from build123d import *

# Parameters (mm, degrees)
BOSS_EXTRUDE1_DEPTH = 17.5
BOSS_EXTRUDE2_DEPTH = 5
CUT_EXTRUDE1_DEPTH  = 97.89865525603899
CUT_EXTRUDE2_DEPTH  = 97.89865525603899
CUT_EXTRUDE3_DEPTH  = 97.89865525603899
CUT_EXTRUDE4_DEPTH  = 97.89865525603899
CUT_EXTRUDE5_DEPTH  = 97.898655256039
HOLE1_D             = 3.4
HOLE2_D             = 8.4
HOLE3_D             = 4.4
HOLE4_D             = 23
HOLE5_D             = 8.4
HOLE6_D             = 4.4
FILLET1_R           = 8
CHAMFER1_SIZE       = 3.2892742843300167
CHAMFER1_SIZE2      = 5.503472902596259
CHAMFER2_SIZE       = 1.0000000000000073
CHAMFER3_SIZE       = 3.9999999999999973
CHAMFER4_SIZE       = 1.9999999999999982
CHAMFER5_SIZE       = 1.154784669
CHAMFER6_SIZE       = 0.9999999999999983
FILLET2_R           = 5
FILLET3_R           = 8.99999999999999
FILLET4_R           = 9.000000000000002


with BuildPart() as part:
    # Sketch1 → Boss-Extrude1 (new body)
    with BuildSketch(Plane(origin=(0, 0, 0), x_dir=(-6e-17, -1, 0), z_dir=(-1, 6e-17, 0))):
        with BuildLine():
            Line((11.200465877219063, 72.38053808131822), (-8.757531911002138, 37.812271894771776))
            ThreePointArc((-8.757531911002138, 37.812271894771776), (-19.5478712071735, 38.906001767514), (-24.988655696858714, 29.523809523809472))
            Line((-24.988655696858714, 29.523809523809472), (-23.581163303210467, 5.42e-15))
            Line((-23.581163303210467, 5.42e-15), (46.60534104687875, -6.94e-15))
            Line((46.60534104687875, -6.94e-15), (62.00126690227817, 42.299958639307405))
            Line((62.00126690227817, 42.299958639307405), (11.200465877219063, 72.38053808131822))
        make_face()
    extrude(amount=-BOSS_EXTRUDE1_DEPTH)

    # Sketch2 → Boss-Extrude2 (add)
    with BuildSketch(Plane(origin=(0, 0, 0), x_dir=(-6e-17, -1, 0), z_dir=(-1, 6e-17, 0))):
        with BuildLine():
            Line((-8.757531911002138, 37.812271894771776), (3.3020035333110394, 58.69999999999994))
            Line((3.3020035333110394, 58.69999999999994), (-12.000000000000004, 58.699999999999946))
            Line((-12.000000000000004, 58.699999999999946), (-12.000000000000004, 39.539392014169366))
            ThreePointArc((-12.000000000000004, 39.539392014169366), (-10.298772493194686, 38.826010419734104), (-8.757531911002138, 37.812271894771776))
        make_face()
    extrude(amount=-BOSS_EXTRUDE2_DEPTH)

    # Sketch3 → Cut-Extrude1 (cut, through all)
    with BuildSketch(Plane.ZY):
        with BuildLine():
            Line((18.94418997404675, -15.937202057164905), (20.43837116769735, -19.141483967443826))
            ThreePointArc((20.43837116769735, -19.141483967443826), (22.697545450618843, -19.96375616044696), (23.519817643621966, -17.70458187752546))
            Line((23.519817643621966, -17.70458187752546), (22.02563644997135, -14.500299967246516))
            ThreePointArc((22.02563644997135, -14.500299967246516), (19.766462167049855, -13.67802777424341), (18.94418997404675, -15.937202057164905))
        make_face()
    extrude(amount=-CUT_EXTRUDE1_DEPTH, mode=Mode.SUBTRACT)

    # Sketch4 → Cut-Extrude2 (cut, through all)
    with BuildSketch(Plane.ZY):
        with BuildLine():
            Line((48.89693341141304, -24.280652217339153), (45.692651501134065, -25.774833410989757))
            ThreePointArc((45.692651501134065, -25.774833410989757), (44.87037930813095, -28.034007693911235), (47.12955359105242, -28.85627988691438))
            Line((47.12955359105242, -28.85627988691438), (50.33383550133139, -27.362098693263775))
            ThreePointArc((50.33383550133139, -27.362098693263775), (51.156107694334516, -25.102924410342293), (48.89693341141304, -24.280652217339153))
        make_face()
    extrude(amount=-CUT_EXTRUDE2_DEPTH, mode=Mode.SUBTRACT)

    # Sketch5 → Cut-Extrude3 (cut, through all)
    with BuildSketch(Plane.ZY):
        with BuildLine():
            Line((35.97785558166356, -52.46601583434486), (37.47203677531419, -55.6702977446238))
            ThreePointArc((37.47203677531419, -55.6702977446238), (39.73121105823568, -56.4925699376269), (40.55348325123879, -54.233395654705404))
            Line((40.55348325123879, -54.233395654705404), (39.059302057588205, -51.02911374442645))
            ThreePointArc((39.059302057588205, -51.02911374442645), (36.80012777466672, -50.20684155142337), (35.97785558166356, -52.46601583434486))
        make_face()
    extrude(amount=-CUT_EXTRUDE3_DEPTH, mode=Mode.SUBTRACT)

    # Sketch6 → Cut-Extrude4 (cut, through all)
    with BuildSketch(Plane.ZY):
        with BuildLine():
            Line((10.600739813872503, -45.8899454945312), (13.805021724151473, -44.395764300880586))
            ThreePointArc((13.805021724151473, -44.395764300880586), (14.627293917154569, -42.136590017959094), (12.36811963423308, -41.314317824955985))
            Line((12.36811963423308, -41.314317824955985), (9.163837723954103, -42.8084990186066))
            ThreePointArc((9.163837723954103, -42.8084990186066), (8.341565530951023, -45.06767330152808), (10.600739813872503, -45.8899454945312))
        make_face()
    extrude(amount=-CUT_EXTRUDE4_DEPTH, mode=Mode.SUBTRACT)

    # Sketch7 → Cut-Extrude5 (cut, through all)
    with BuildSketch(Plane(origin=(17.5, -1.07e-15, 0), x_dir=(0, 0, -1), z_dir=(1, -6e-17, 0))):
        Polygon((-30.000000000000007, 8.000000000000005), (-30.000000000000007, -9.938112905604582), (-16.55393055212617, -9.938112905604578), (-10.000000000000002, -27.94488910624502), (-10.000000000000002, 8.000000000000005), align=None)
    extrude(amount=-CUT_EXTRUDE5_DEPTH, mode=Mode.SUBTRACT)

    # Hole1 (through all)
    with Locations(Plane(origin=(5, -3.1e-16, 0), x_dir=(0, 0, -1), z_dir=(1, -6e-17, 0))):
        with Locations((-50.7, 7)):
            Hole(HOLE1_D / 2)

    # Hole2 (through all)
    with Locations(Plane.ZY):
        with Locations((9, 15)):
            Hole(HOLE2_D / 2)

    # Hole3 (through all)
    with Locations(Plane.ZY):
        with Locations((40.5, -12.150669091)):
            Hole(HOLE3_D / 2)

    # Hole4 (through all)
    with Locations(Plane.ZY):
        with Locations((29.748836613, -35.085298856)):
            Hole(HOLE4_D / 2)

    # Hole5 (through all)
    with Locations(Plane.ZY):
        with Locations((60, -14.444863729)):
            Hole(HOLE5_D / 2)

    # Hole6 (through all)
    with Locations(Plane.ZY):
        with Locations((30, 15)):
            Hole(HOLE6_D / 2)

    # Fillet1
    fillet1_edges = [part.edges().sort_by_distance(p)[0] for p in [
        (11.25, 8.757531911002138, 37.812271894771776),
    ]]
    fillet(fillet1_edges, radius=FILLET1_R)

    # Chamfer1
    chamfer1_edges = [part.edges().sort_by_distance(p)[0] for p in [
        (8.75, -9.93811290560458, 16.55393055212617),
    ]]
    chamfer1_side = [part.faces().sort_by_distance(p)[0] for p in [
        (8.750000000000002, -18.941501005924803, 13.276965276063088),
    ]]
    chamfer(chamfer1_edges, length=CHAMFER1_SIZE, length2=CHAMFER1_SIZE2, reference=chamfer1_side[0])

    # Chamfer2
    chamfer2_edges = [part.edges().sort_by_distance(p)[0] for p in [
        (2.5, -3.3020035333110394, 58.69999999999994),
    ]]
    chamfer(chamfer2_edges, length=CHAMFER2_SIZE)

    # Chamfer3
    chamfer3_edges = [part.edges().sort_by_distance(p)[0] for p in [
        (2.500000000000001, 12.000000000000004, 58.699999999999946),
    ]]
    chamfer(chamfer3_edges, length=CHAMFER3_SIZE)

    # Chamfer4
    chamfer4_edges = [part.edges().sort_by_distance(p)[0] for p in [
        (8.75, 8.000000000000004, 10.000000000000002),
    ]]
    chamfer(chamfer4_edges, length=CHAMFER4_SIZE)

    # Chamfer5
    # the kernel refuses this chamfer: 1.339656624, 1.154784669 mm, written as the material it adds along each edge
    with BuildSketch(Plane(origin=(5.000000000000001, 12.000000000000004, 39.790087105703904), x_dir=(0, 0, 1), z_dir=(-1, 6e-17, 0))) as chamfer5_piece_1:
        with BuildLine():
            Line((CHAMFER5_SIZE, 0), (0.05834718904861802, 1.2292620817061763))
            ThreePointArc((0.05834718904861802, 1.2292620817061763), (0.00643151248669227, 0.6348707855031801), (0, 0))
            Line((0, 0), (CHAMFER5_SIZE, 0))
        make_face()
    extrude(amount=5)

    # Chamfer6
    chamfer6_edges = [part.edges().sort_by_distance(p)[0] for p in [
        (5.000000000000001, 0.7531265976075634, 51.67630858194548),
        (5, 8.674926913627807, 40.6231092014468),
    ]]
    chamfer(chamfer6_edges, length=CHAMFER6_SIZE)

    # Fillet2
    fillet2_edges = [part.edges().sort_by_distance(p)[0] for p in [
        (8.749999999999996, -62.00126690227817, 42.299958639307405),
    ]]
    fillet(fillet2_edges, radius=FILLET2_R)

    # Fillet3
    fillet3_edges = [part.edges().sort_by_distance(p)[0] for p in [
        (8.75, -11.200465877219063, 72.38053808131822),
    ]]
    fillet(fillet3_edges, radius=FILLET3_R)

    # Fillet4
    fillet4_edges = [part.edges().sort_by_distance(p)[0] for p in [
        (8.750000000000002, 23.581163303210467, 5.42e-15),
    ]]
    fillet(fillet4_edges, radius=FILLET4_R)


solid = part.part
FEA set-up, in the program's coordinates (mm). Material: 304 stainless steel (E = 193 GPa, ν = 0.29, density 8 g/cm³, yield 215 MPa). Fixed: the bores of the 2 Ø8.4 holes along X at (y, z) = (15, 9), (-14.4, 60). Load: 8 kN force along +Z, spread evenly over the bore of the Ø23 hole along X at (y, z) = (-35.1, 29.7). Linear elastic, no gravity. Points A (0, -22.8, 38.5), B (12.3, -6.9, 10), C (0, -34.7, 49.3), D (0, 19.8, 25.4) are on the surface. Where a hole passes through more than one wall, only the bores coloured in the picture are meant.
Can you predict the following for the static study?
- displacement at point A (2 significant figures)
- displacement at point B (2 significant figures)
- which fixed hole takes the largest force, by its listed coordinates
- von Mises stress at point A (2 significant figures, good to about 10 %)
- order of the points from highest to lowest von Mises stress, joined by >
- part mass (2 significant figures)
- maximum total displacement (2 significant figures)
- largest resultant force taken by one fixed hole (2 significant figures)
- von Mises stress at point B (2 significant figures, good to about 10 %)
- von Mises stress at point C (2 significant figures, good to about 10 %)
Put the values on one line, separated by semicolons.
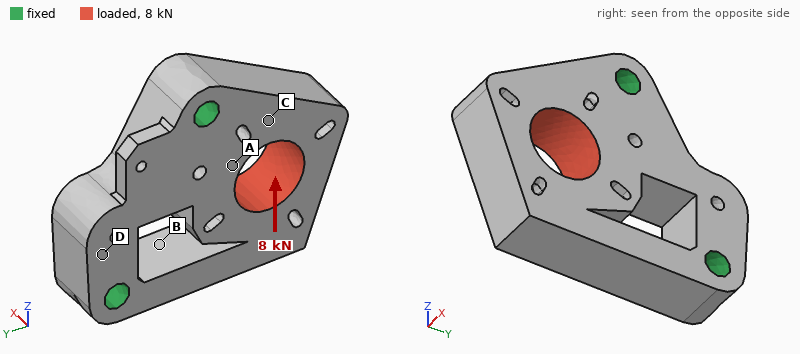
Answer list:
3.5 µm; 3.0 µm; (-14.4, 60); 28 MPa; A > C > B > D; 450 g; 10 µm; 8.2 kN; 12 MPa; 19 MPa
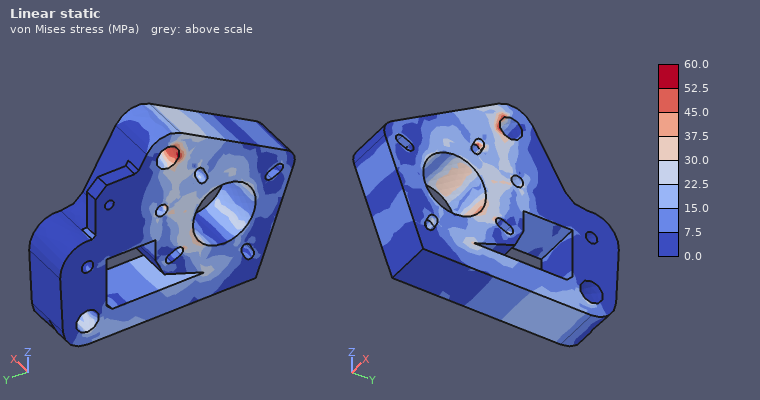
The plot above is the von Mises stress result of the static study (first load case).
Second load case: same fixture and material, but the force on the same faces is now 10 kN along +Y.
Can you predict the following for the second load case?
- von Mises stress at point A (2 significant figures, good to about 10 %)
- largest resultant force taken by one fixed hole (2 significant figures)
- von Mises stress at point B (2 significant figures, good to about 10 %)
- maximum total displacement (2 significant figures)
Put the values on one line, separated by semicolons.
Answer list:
12 MPa; 5.2 kN; 30 MPa; 9.3 µm
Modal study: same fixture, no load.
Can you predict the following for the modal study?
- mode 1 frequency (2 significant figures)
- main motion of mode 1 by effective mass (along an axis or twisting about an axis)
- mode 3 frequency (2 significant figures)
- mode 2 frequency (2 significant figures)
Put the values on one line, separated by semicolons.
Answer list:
4000 Hz; along X; 9500 Hz; 8700 Hz
